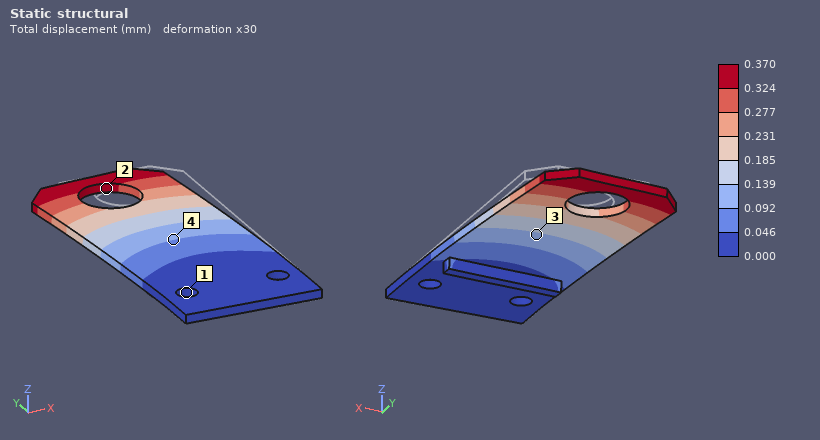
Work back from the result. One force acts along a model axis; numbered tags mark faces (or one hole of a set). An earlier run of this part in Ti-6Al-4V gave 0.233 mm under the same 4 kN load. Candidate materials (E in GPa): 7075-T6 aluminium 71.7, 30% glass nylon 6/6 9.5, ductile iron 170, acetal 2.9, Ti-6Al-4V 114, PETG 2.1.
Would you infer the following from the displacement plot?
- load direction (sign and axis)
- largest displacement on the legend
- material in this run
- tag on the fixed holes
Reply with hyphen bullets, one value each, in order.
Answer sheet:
- -X
- 0.370 mm
- 7075-T6 aluminium
- 1
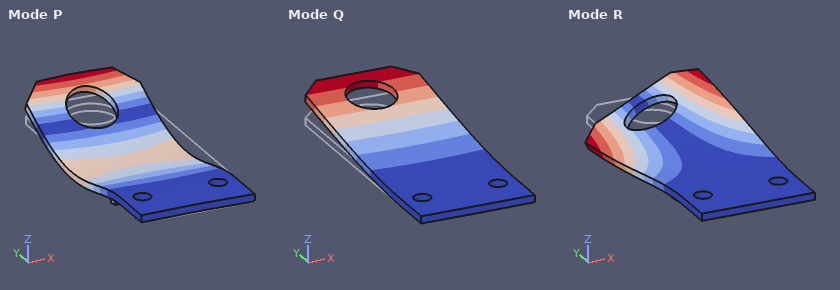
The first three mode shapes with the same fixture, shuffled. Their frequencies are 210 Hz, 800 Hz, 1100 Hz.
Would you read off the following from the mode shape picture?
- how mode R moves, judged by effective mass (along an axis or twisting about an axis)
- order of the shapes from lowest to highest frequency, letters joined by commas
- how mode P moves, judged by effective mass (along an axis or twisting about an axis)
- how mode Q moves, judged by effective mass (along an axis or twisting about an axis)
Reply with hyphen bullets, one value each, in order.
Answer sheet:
- twisting about Y
- Q, R, P
- along Z
- along Z
